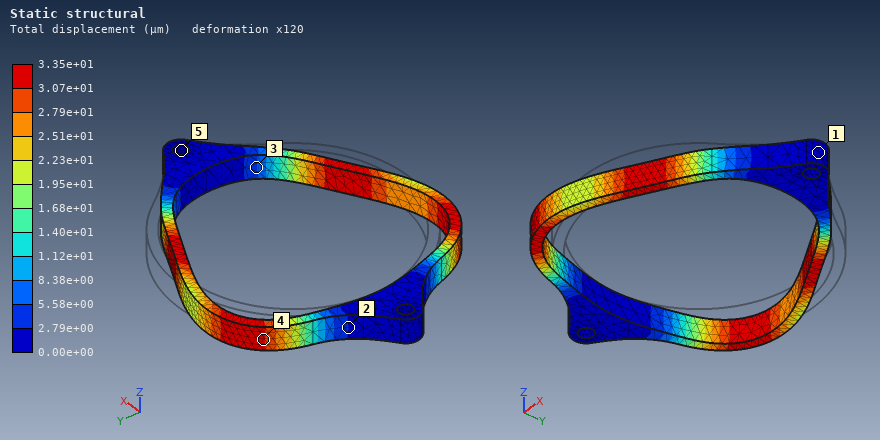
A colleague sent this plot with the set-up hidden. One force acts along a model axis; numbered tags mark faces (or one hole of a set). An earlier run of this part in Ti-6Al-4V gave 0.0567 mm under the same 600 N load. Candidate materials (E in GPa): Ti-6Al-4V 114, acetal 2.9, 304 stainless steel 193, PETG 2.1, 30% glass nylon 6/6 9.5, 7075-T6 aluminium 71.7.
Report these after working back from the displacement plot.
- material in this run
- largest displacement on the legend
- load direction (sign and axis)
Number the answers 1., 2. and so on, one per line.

1. 304 stainless steel
2. 3.35e+01 µm
3. -X
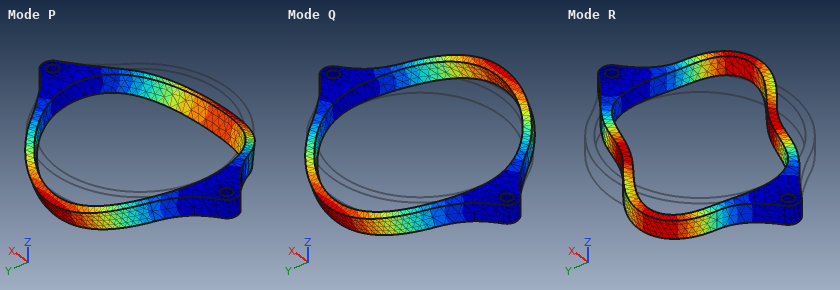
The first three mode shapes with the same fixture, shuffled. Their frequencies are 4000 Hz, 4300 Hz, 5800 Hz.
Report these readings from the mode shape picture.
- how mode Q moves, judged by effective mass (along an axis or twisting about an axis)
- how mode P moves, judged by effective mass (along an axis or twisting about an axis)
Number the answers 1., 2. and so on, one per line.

1. twisting about X
2. along Z
